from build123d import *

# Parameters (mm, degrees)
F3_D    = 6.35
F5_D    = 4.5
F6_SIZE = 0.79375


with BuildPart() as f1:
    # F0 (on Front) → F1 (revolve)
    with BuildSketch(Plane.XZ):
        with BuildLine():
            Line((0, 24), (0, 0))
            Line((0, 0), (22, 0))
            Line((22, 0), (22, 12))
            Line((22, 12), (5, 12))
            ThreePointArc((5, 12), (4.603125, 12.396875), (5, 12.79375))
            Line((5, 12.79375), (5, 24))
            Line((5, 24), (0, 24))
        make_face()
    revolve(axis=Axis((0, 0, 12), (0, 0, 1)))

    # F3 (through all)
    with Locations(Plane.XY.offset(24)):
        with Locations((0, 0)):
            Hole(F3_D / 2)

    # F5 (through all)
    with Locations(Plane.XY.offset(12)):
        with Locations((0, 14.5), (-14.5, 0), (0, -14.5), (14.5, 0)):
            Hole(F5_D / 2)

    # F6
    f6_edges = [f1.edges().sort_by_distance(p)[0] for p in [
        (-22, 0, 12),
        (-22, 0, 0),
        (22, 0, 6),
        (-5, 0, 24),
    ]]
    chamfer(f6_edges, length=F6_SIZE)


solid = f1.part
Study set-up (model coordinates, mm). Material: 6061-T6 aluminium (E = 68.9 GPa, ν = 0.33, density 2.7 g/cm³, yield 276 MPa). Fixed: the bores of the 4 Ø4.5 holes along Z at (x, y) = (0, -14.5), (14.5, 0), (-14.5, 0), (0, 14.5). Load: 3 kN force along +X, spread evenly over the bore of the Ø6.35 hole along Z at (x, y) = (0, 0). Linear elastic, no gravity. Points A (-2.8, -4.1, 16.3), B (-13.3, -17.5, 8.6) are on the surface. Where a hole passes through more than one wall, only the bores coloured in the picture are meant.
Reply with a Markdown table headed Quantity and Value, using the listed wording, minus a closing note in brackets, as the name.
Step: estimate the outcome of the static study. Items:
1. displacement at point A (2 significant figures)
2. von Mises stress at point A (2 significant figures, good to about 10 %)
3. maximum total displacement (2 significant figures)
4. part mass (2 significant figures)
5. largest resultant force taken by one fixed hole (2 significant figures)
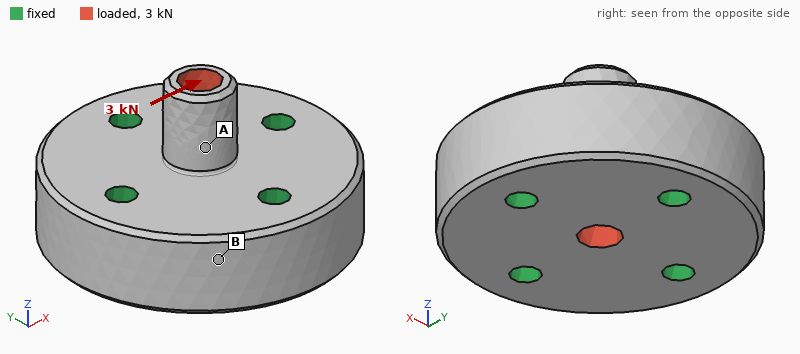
| Quantity | Value |
|---|---|
| displacement at point A | 20 µm |
| von Mises stress at point A | 51 MPa |
| maximum total displacement | 45 µm |
| part mass | 47 g |
| largest resultant force taken by one fixed hole | 1.2 kN |
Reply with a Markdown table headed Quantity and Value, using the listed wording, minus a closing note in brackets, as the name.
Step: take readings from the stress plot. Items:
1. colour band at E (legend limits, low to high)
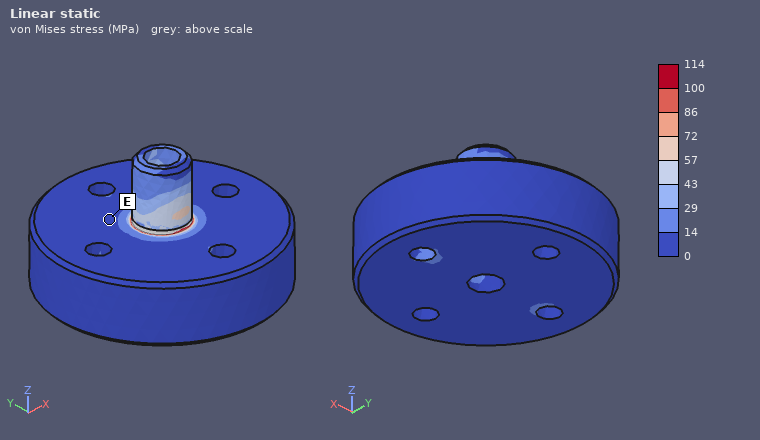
| Quantity | Value |
|---|---|
| colour band at E | 0 to 14 MPa |
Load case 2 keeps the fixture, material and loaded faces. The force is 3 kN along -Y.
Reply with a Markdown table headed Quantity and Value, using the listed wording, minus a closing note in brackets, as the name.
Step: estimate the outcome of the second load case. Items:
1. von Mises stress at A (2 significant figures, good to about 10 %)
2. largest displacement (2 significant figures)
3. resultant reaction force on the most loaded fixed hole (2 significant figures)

| Quantity | Value |
|---|---|
| von Mises stress at A | 44 MPa |
| largest displacement | 45 µm |
| resultant reaction force on the most loaded fixed hole | 1.2 kN |
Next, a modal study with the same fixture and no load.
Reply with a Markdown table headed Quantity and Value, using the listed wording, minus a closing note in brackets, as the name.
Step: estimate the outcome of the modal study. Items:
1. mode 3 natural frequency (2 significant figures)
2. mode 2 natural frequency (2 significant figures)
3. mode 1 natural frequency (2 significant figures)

| Quantity | Value |
|---|---|
| mode 3 natural frequency | 46 kHz |
| mode 2 natural frequency | 28 kHz |
| mode 1 natural frequency | 28 kHz |
